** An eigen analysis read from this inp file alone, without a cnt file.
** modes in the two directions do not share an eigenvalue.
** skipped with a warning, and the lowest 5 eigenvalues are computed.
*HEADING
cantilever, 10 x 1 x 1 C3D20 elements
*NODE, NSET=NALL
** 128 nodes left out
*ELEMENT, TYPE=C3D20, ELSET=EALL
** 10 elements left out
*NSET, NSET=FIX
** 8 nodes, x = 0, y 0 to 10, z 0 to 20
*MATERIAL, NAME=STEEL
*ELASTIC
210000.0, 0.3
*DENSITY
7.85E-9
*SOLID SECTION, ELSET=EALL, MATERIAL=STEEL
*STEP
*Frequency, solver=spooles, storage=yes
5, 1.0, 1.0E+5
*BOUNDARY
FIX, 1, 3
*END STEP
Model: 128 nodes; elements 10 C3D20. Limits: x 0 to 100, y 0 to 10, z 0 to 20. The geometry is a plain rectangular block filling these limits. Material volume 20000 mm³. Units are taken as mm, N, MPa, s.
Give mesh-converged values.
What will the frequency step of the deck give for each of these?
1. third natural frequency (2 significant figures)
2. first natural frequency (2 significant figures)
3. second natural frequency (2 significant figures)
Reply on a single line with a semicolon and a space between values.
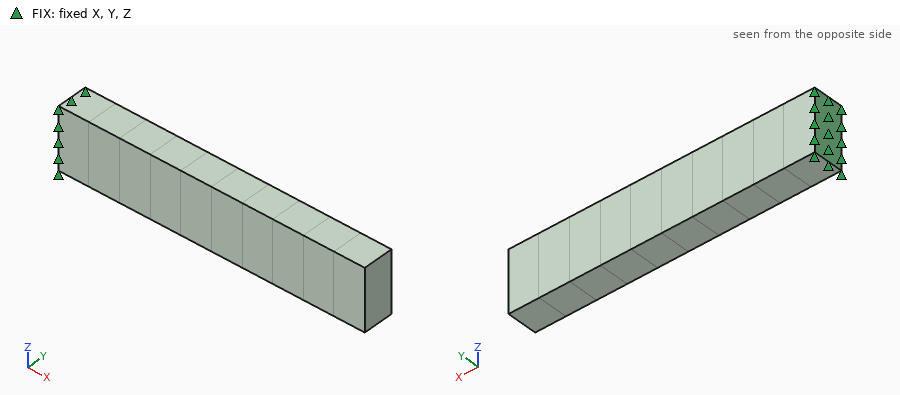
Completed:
5000 Hz; 840 Hz; 1600 Hz
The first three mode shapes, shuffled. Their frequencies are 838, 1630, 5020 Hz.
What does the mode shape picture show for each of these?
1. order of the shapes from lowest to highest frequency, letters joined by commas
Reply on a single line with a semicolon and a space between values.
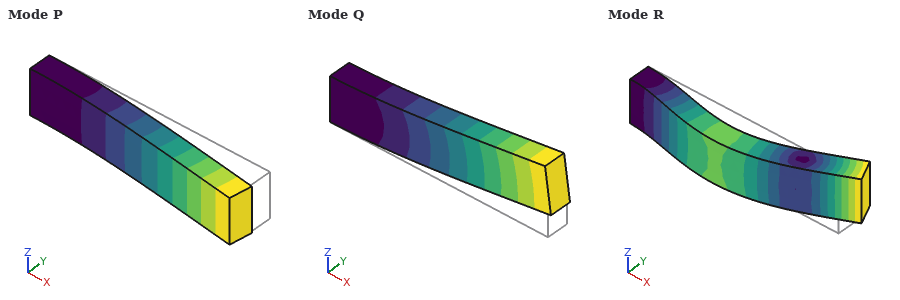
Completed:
P, Q, R
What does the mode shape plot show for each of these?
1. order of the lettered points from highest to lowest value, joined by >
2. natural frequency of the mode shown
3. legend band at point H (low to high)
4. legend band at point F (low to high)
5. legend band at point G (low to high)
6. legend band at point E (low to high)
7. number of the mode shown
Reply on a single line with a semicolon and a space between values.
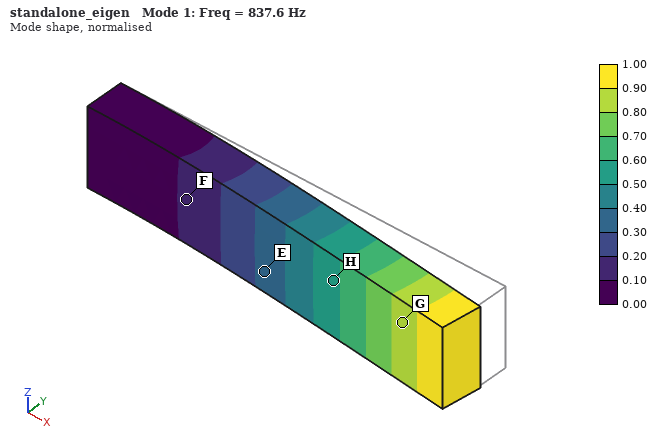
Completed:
G > H > E > F; 837.6 Hz; 0.50 to 0.60; 0.10 to 0.20; 0.80 to 0.90; 0.30 to 0.40; 1
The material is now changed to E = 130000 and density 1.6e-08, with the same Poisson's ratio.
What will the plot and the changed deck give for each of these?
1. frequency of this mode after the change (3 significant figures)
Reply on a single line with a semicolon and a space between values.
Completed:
462 Hz
